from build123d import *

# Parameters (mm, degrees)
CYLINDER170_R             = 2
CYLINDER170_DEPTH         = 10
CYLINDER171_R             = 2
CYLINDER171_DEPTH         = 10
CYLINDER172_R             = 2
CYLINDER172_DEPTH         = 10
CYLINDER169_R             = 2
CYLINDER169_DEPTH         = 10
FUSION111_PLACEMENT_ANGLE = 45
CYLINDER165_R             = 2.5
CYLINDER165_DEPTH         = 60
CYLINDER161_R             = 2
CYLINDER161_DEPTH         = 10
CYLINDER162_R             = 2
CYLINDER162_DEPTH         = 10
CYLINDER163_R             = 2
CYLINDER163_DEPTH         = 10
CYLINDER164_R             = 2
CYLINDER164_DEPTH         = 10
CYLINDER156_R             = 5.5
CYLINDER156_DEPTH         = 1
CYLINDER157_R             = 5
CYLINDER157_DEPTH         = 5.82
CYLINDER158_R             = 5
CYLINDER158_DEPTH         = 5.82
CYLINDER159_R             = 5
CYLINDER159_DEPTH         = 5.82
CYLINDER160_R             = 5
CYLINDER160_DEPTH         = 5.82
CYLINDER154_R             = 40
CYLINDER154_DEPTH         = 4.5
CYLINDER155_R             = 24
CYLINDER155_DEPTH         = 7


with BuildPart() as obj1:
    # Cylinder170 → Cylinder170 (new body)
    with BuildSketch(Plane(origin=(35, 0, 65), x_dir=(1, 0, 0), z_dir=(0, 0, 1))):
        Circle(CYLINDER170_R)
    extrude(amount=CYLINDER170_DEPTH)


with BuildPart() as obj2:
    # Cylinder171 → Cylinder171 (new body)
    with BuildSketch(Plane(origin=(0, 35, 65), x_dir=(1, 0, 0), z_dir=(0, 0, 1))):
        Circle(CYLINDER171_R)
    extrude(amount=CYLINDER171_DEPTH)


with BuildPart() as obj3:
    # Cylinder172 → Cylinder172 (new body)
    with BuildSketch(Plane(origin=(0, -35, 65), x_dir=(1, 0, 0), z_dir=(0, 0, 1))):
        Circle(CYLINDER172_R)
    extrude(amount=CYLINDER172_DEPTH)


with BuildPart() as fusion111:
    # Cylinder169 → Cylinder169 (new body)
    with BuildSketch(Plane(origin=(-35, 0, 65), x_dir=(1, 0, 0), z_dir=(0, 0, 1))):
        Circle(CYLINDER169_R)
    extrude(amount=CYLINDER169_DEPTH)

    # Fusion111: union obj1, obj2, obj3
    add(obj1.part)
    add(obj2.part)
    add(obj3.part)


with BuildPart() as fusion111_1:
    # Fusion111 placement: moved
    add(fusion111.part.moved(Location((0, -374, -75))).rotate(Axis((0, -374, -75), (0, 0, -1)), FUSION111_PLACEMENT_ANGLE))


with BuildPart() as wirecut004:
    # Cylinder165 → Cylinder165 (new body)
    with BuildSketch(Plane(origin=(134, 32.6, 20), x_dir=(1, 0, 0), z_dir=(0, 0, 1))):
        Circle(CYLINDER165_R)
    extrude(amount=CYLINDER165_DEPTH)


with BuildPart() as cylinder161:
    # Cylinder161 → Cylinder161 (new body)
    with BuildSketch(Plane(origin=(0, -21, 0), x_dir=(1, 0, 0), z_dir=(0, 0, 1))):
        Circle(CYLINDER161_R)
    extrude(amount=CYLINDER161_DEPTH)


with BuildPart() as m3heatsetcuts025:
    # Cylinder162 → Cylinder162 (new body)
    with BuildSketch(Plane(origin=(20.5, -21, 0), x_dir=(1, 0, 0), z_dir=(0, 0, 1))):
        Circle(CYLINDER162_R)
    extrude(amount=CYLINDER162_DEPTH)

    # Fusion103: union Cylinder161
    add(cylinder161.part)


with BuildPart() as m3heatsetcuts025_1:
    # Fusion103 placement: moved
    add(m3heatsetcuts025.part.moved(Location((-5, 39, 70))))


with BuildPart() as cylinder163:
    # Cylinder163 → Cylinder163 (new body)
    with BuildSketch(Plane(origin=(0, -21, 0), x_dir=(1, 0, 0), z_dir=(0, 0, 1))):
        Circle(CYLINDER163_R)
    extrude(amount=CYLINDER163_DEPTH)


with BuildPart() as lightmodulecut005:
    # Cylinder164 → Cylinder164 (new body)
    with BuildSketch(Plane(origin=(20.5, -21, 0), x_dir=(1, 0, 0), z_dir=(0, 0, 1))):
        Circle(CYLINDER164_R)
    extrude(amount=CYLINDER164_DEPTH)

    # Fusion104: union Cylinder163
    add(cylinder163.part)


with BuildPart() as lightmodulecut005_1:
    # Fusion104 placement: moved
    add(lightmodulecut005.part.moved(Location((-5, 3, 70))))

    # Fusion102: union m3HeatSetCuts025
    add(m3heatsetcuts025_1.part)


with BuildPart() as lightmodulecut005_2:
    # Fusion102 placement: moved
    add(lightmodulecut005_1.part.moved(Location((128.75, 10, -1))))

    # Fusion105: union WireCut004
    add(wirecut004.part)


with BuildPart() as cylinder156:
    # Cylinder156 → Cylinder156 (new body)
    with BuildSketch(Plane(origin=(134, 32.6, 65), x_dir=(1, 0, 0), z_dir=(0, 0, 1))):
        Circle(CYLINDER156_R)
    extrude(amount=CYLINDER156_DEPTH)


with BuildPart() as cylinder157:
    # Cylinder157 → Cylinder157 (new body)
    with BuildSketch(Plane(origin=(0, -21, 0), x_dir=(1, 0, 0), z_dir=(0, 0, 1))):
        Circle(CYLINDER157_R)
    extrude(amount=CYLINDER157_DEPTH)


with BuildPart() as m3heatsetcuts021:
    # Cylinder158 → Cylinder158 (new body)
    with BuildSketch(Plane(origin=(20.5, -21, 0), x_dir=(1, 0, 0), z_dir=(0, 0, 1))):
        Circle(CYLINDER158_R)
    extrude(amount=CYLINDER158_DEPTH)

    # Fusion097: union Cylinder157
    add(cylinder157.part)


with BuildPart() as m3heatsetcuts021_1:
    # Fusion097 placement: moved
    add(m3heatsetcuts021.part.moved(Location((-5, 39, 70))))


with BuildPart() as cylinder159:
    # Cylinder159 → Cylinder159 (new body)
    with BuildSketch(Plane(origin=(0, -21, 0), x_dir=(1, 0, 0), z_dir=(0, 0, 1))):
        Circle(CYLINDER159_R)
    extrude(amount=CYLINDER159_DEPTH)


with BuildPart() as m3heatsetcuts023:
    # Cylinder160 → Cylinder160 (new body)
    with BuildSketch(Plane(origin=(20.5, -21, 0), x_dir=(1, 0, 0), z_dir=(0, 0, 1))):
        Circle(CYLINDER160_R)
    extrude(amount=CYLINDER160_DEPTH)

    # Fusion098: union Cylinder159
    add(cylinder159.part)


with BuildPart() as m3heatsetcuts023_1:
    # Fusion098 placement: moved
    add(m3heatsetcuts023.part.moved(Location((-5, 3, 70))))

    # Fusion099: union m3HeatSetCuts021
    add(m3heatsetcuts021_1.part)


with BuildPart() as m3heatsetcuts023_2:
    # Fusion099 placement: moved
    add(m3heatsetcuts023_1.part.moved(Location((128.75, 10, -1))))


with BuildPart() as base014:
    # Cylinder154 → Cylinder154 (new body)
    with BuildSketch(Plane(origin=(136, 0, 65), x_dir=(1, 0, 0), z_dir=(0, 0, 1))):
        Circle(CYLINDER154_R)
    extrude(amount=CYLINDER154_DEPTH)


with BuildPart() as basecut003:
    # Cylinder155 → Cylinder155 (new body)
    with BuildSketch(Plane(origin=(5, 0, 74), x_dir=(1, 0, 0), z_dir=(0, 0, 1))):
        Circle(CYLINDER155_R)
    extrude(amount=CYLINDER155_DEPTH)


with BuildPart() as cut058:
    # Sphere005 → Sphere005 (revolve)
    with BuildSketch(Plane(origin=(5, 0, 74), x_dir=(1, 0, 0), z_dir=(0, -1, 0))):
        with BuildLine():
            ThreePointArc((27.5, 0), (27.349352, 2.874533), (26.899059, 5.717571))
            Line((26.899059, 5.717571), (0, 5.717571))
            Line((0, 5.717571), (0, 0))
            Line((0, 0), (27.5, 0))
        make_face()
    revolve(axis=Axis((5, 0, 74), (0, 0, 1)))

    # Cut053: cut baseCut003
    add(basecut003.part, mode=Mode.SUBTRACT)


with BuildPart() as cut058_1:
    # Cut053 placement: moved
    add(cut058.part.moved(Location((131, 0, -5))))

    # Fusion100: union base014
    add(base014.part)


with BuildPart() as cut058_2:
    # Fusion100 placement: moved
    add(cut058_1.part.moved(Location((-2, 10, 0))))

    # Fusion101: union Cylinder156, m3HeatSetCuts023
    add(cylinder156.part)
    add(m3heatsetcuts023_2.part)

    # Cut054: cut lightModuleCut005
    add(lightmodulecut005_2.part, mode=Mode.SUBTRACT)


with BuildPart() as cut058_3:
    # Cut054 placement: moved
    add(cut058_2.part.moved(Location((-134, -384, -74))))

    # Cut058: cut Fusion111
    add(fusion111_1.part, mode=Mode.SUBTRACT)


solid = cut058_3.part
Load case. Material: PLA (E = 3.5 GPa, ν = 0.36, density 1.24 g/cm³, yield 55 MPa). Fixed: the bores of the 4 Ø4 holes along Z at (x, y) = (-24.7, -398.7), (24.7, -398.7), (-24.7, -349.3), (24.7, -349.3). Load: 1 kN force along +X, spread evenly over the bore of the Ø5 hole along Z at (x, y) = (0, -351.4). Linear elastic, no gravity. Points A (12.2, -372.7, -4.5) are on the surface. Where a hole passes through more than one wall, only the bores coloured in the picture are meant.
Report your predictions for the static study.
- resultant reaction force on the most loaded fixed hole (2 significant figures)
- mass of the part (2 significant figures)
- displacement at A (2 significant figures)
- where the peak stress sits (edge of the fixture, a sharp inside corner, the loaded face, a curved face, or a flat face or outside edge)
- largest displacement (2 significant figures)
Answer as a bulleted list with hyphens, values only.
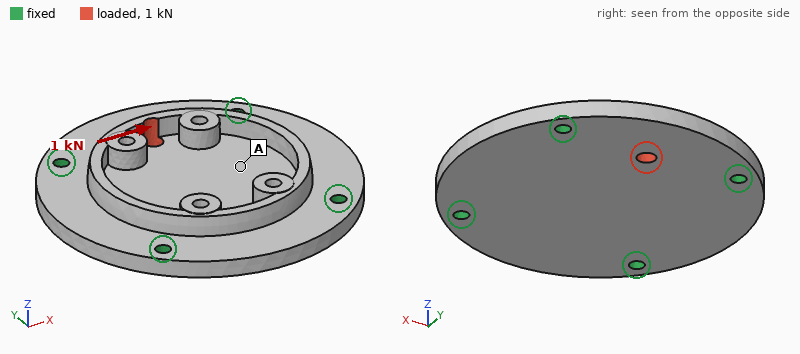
- 440 N
- 33 g
- 14 µm
- the loaded face
- 60 µm
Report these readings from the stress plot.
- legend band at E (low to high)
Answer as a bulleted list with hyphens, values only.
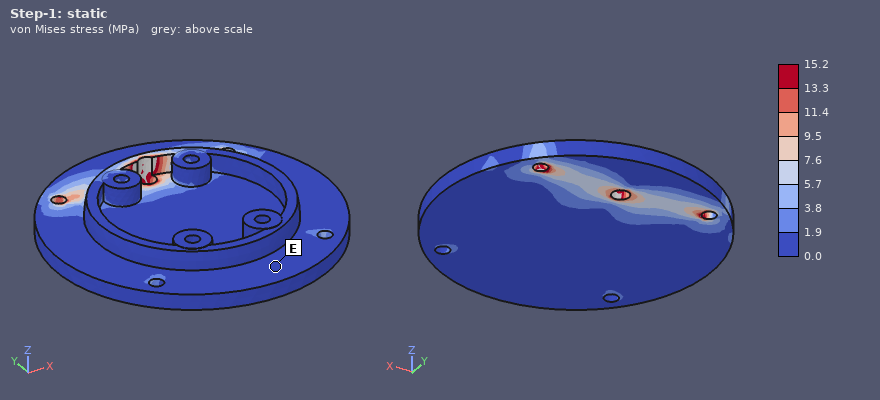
- 0.0 to 1.9 MPa
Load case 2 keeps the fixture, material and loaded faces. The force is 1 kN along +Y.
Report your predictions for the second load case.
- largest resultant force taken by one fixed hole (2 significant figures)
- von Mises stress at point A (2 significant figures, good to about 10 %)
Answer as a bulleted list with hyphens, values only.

- 300 N
- 3.7 MPa
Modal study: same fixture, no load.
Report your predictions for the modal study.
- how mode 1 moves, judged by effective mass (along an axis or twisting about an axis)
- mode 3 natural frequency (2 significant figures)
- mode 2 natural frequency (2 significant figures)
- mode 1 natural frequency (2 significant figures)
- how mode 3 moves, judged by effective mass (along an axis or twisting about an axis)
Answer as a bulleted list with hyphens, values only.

- along Z
- 2900 Hz
- 2700 Hz
- 2400 Hz
- twisting about X
